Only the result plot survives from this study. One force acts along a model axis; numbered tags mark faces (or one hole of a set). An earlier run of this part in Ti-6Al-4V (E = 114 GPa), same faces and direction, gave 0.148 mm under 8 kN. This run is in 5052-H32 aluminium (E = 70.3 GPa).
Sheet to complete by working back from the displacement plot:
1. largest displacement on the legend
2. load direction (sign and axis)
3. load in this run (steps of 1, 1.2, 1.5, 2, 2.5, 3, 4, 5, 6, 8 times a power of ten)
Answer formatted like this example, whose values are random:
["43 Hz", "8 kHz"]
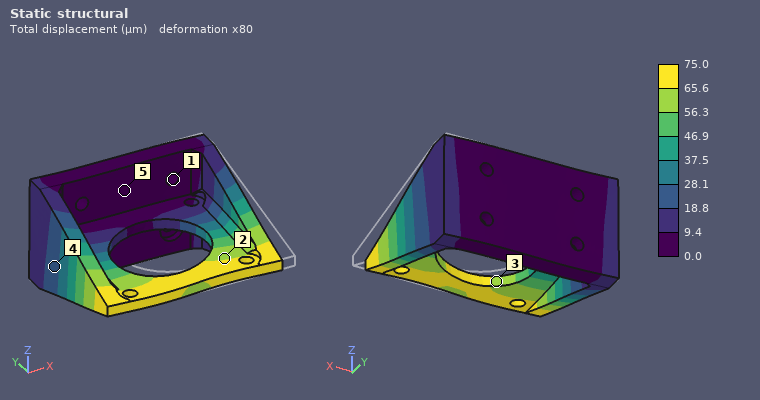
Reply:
["75.0 µm", "-X", "2.5 kN"]
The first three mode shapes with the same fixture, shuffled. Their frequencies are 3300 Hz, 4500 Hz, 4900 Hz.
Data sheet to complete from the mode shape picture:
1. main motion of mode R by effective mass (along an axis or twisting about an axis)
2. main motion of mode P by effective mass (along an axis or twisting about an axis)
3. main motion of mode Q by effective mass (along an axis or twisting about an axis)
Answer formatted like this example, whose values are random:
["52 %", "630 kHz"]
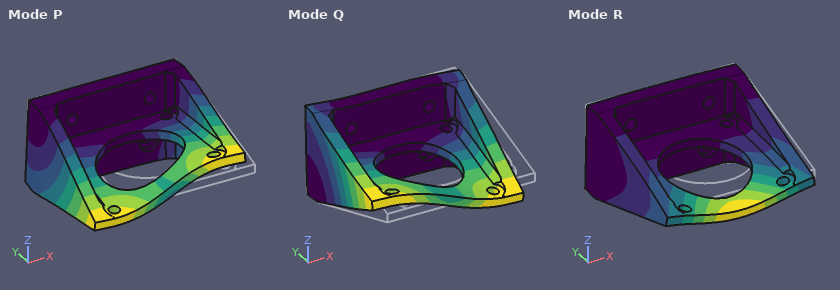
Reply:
["along Z", "along X", "along X"]
